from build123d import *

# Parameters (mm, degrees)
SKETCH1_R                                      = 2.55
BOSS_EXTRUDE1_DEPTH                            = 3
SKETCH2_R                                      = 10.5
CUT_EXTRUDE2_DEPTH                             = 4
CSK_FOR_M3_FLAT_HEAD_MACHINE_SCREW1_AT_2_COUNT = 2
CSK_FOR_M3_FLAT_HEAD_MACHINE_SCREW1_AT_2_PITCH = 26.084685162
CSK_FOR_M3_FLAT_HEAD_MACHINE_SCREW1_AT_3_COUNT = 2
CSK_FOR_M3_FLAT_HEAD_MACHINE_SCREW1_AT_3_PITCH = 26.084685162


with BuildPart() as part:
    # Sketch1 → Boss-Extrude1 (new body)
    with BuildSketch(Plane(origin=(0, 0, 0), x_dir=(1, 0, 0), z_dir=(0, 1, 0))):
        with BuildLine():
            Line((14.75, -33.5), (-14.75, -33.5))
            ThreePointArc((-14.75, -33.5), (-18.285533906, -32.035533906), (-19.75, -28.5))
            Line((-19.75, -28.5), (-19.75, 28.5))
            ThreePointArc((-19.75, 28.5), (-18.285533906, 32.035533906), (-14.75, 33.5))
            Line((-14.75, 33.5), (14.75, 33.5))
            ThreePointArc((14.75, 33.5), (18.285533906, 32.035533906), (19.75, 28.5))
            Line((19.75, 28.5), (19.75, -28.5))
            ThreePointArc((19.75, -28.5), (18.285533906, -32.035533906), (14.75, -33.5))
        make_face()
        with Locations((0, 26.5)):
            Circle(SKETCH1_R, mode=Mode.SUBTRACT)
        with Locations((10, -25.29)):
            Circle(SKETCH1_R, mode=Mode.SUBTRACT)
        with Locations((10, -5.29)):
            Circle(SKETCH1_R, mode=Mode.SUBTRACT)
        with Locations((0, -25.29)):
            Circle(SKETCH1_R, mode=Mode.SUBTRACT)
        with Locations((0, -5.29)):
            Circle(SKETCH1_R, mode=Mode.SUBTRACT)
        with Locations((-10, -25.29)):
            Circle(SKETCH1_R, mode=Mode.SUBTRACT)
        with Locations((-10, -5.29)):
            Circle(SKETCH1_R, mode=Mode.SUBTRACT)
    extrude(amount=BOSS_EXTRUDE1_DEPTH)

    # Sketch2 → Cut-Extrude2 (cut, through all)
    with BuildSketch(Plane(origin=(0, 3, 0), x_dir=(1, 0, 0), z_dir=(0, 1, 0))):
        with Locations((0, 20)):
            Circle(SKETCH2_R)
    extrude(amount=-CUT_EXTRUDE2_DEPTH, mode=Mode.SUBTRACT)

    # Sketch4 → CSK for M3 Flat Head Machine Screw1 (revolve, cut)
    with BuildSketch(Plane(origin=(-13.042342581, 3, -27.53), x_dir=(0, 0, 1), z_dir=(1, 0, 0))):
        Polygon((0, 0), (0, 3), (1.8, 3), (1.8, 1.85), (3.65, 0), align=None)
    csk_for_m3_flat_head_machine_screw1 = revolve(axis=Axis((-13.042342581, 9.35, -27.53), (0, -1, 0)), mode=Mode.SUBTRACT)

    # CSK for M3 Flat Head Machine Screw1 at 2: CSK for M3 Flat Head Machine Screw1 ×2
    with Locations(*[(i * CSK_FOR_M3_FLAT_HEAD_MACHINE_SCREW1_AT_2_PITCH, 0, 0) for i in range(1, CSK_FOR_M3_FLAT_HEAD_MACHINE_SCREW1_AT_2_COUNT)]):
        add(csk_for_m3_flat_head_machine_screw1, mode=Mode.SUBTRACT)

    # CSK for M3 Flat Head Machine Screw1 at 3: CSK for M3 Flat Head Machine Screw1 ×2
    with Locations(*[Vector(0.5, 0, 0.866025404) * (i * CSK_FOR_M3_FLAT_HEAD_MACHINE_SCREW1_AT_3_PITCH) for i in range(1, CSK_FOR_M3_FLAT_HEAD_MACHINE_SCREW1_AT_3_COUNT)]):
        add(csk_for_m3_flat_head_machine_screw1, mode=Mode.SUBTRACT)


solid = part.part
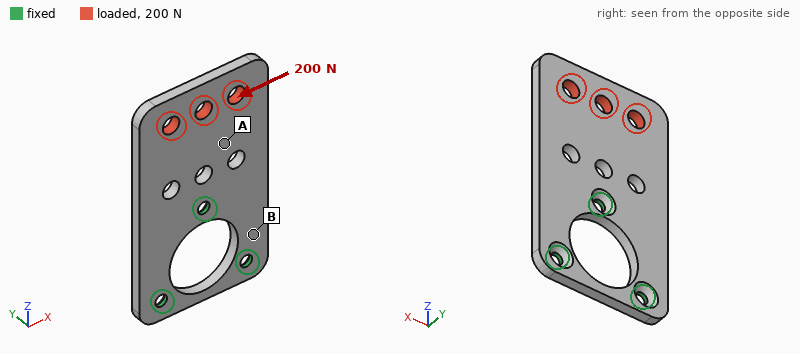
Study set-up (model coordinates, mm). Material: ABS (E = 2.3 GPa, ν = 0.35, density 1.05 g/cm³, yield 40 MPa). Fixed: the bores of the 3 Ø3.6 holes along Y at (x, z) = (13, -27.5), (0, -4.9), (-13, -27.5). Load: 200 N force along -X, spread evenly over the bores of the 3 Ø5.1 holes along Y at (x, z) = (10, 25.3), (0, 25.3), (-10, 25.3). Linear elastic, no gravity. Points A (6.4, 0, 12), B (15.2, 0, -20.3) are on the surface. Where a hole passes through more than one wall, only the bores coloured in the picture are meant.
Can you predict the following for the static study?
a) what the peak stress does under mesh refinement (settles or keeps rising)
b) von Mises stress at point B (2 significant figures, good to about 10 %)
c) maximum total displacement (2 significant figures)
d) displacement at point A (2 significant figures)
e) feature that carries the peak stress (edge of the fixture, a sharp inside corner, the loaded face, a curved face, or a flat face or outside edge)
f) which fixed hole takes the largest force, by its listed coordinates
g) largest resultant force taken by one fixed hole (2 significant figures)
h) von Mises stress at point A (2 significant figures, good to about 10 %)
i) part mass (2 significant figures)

keeps rising
9.2 MPa
0.42 mm
0.18 mm
edge of the fixture
(0, -4.9)
260 N
2.6 MPa
6.6 g
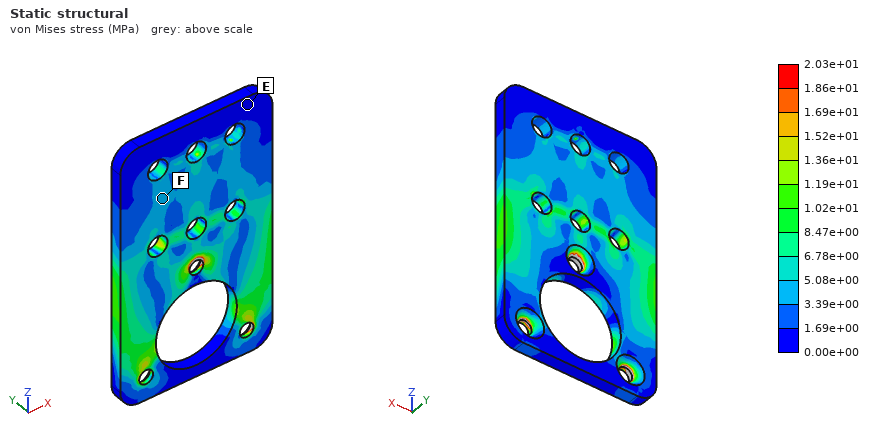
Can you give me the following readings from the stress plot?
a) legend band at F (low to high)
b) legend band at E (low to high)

3.39e+00 to 5.08e+00 MPa
0.00e+00 to 1.69e+00 MPa
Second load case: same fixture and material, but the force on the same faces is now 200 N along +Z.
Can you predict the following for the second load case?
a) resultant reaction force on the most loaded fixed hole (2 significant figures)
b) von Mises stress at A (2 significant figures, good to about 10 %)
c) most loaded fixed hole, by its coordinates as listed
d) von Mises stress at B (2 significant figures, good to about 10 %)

110 N
2.7 MPa
(0, -4.9)
2.0 MPa
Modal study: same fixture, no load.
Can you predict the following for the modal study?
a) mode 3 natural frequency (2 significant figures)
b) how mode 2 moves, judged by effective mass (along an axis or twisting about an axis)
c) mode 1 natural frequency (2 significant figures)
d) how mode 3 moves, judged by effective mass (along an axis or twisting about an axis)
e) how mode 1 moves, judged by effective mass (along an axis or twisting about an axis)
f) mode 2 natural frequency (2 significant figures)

1700 Hz
twisting about Z
390 Hz
along Y
along Y
670 Hz
